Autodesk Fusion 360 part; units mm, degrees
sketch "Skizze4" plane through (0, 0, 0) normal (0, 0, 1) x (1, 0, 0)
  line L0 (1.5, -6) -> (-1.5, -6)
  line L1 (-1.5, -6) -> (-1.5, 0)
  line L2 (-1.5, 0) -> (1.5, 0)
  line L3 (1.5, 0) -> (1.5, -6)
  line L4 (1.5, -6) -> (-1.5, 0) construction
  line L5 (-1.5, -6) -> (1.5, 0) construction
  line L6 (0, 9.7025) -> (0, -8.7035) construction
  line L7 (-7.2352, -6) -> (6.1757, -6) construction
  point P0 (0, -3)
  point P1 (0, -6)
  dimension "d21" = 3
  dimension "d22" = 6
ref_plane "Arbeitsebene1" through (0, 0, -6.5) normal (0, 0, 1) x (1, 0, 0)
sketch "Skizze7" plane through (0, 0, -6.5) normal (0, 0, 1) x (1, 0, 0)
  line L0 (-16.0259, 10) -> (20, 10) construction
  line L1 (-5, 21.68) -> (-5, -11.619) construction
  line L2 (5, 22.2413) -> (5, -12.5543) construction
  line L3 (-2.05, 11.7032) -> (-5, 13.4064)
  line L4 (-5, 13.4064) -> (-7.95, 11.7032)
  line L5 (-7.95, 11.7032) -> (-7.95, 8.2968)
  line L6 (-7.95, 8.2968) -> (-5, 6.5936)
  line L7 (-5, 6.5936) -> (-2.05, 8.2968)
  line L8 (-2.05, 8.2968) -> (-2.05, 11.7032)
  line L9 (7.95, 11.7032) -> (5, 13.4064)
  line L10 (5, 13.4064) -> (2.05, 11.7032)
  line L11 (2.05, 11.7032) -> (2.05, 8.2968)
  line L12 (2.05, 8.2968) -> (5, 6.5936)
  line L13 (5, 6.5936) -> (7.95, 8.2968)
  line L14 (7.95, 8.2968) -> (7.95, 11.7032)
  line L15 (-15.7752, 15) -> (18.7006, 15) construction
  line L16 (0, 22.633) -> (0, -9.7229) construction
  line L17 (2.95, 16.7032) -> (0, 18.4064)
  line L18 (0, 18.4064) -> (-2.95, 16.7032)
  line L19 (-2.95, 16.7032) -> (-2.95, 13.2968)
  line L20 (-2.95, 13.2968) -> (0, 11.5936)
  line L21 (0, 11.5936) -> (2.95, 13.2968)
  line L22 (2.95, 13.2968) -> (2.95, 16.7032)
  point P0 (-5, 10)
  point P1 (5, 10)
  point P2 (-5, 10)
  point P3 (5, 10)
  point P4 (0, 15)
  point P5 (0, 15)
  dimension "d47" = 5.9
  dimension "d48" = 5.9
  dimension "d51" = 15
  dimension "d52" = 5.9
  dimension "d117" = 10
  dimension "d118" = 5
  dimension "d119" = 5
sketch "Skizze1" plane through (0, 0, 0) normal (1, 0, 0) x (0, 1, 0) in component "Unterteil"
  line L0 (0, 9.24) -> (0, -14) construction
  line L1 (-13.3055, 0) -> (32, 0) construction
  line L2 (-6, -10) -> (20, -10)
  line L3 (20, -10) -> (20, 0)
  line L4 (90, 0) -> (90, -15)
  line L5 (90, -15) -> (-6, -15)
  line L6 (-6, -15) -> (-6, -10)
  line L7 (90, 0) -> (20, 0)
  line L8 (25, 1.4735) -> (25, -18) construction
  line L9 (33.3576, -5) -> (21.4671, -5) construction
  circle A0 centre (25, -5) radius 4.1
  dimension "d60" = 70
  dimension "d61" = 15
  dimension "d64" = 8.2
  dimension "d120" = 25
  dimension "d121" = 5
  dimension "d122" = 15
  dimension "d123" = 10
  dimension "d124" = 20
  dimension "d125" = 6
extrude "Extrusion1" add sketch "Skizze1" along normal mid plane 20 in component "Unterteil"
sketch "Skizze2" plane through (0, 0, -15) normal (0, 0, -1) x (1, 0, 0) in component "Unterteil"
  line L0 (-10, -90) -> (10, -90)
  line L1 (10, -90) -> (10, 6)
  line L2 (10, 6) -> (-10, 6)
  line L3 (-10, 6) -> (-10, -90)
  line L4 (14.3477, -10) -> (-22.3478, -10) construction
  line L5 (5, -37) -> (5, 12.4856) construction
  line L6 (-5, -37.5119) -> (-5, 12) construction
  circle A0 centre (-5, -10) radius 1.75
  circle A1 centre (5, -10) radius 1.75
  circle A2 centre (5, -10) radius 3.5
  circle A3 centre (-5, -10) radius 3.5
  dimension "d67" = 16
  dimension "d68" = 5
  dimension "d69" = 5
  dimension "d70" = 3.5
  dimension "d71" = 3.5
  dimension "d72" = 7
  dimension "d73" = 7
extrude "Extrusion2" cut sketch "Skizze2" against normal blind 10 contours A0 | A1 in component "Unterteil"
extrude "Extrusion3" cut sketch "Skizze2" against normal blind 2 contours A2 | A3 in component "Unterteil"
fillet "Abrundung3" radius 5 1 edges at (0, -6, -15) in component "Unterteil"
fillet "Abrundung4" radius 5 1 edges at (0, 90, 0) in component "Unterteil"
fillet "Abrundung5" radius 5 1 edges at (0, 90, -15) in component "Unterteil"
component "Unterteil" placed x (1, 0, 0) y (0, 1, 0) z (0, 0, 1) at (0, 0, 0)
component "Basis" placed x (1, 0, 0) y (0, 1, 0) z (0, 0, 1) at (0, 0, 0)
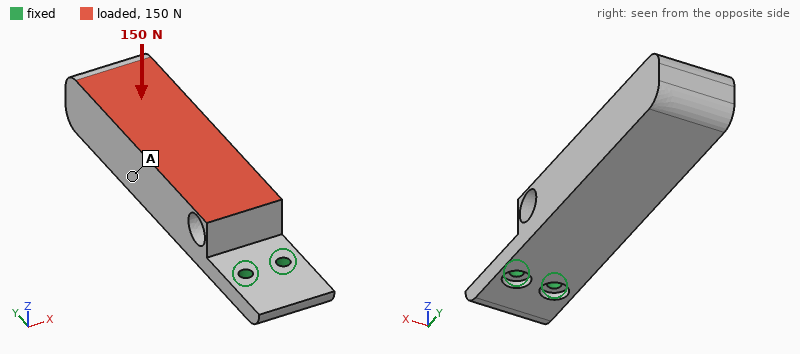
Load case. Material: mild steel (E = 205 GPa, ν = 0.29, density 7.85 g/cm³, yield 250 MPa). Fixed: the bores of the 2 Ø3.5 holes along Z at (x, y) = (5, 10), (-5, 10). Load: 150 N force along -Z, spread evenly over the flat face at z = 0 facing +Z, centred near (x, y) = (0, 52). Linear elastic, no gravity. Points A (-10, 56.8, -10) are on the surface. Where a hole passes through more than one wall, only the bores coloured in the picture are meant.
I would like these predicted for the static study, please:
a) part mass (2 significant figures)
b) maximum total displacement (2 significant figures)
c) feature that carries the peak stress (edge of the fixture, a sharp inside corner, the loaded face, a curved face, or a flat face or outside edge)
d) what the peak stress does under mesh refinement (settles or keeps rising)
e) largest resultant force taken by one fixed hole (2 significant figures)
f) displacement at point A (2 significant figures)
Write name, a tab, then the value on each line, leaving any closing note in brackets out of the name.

part mass	170 g
maximum total displacement	0.19 mm
feature that carries the peak stress	edge of the fixture
what the peak stress does under mesh refinement	keeps rising
largest resultant force taken by one fixed hole	82 N
displacement at point A	0.10 mm
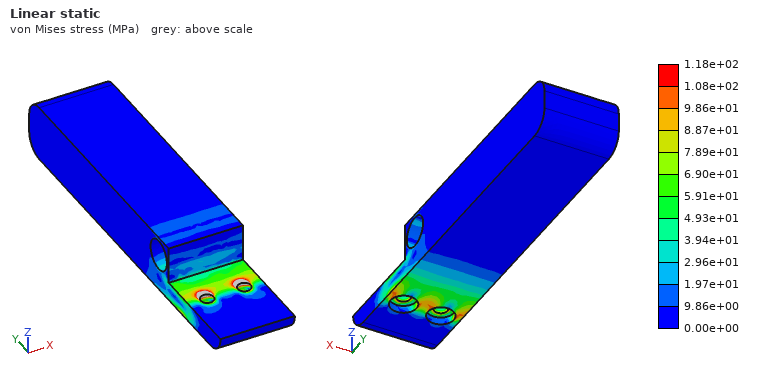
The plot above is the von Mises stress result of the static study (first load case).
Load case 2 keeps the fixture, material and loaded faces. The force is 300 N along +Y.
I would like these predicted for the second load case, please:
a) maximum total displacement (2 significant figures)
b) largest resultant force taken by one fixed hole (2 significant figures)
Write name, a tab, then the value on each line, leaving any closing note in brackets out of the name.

maximum total displacement	0.12 mm
largest resultant force taken by one fixed hole	150 N
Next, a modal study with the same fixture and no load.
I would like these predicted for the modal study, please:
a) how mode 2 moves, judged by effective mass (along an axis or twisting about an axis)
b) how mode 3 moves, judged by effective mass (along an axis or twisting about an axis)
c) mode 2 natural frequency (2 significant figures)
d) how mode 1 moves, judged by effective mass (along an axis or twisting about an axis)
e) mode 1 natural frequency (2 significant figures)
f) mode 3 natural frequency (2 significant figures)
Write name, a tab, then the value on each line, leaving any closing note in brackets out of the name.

how mode 2 moves, judged by effective mass	along X
how mode 3 moves, judged by effective mass	twisting about Y
mode 2 natural frequency	1400 Hz
how mode 1 moves, judged by effective mass	along Z
mode 1 natural frequency	420 Hz
mode 3 natural frequency	4000 Hz
